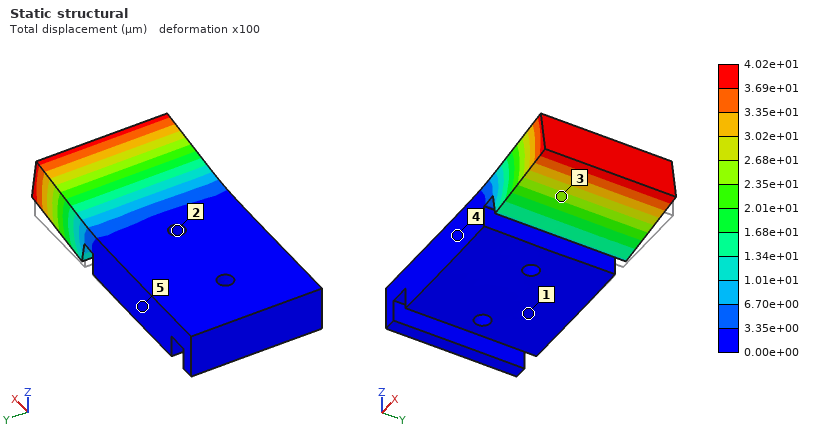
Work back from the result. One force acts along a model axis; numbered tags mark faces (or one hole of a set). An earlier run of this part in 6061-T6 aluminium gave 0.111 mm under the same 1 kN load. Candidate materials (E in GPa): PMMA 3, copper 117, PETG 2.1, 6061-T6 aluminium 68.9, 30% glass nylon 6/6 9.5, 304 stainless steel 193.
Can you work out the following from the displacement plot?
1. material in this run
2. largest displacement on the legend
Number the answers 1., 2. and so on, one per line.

1. 304 stainless steel
2. 4.02e+01 µm
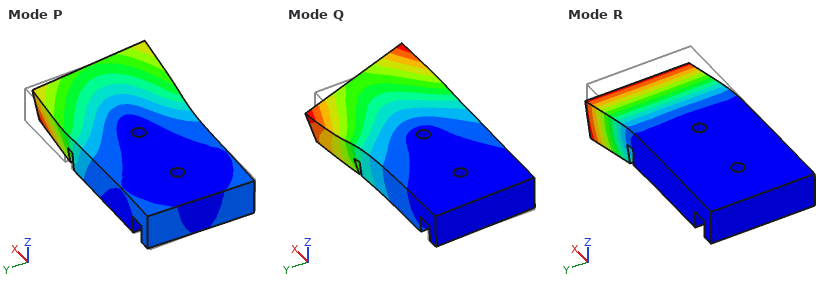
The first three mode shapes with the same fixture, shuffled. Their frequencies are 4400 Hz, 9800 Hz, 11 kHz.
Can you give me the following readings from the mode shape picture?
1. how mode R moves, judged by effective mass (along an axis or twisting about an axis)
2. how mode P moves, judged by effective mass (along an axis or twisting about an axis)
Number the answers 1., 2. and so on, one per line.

1. along Z
2. along Y
